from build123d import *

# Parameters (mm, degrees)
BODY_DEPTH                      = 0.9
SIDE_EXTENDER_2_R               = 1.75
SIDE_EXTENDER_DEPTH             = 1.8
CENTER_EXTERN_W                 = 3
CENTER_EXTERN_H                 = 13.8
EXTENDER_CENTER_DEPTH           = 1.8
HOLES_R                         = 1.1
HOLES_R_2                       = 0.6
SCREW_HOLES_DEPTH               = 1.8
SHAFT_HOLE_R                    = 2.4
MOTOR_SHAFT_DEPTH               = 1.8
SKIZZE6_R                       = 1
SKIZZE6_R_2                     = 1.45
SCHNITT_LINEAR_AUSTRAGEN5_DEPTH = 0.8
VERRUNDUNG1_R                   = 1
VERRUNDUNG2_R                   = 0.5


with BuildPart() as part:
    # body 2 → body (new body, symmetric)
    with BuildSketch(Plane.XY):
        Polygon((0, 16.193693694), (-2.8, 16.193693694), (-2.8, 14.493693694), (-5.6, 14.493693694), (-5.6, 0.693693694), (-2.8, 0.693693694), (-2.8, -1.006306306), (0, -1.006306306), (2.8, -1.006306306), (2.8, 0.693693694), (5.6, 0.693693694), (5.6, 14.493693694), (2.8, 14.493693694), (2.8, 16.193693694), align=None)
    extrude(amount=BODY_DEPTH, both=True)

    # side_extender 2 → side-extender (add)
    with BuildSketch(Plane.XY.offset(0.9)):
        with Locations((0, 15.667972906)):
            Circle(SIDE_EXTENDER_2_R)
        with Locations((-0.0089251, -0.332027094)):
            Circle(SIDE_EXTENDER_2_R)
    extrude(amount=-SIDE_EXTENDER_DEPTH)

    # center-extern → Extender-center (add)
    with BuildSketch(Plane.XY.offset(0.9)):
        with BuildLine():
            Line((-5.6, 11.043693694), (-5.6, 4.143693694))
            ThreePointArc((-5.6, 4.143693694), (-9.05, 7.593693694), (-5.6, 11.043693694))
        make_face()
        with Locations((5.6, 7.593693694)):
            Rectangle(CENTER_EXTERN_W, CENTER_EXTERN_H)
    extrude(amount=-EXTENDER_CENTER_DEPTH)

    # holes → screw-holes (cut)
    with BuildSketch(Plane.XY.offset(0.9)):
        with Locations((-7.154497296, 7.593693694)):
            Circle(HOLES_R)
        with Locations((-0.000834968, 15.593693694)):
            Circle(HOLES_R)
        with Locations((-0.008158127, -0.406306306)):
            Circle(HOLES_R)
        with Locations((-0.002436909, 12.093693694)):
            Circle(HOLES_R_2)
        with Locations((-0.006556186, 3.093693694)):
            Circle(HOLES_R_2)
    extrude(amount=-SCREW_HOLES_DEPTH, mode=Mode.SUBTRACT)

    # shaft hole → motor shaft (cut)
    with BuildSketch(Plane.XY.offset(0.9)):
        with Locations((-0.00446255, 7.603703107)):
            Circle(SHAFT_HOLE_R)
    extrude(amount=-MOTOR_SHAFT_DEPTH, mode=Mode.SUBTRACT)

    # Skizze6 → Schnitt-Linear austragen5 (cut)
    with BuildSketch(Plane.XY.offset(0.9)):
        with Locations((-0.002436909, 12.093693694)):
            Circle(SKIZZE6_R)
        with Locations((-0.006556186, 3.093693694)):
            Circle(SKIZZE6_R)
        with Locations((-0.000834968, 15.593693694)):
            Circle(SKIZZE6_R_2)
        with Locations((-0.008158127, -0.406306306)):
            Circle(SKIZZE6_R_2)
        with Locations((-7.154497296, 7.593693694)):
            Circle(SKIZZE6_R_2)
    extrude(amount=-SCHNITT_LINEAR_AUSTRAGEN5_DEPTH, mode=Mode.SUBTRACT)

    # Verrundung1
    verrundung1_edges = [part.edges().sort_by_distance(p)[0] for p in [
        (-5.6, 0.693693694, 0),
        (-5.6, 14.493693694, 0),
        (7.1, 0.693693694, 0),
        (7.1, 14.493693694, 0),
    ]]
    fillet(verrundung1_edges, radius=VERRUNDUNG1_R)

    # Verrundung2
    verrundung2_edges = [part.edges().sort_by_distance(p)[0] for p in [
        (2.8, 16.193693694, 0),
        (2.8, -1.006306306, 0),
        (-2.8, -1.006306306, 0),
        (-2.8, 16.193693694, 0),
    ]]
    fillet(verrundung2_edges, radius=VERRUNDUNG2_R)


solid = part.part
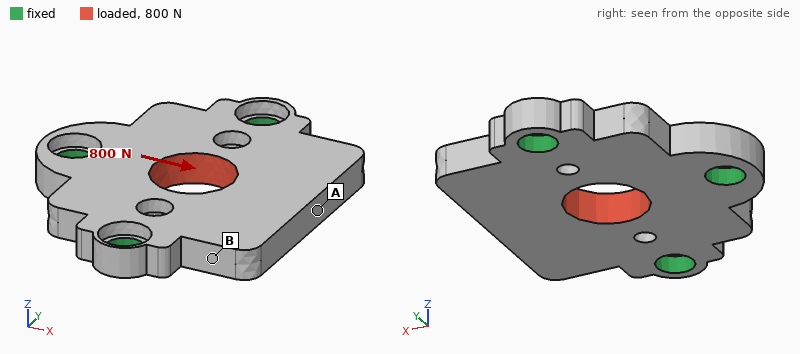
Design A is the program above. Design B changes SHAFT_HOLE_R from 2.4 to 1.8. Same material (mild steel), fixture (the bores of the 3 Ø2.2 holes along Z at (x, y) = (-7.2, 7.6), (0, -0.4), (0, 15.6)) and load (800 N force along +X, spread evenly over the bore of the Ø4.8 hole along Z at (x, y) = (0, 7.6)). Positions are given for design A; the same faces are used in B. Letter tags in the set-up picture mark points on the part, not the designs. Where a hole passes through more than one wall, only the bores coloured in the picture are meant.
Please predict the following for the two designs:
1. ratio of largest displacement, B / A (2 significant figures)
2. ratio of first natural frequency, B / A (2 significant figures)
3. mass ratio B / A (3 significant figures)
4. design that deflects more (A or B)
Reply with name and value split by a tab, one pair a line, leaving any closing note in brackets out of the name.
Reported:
ratio of largest displacement, B / A	0.89
ratio of first natural frequency, B / A	1.0
mass ratio B / A	1.04
design that deflects more	A
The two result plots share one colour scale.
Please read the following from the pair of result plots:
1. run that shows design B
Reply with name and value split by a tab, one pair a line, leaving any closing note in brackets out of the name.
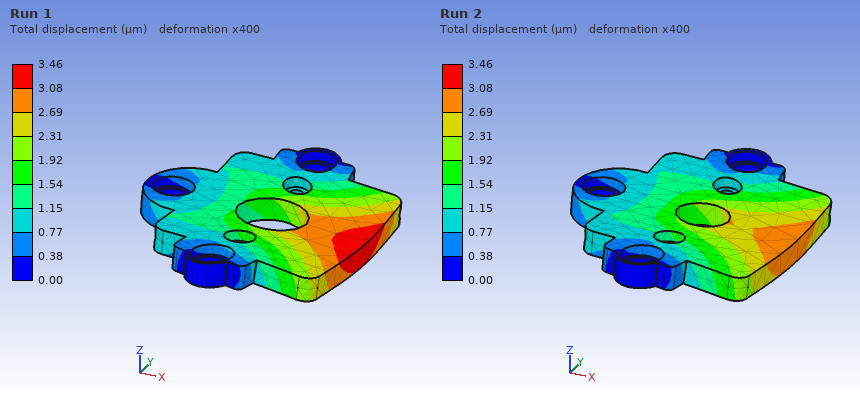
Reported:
run that shows design B	Run 2
